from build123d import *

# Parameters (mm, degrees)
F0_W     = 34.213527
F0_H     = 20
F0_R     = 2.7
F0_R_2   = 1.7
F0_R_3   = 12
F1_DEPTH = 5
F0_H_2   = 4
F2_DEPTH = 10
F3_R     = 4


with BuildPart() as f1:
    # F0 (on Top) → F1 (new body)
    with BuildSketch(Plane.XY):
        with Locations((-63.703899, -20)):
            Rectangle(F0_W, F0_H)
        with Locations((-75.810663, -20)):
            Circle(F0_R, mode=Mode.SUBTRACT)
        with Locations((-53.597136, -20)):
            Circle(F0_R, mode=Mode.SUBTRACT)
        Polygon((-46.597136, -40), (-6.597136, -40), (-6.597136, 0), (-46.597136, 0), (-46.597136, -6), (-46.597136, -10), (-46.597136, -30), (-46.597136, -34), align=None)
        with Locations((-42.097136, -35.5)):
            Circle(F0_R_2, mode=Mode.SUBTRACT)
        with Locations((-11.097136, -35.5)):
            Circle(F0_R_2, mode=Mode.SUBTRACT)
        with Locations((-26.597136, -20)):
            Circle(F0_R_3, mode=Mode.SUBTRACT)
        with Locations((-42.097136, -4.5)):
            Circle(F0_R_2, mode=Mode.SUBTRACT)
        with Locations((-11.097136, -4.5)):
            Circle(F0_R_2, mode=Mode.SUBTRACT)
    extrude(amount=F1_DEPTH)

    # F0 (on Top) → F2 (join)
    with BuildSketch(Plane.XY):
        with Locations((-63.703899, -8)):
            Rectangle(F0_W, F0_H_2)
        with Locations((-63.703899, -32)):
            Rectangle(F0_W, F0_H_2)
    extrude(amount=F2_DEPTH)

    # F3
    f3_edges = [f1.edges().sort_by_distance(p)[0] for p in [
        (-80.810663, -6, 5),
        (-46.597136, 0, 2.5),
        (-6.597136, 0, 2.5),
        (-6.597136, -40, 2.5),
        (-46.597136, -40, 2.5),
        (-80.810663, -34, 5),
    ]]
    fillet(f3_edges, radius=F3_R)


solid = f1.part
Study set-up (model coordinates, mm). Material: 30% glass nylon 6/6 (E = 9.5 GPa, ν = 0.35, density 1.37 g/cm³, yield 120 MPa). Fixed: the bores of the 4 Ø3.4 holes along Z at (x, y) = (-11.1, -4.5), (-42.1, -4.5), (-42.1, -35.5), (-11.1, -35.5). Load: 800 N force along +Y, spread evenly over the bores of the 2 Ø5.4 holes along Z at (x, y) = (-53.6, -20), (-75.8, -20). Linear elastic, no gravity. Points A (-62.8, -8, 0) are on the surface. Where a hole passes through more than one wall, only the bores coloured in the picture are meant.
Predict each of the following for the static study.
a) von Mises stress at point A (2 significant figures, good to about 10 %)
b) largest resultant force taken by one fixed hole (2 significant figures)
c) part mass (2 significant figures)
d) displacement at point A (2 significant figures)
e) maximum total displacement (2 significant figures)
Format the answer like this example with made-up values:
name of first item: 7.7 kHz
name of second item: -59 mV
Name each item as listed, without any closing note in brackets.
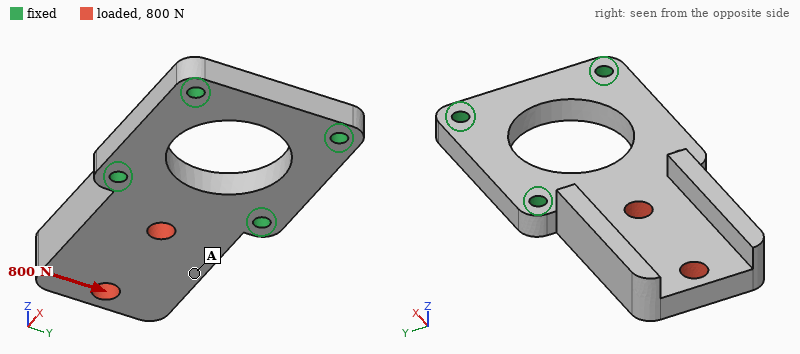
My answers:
von Mises stress at point A: 5.9 MPa
largest resultant force taken by one fixed hole: 710 N
part mass: 16 g
displacement at point A: 0.070 mm
maximum total displacement: 0.12 mm
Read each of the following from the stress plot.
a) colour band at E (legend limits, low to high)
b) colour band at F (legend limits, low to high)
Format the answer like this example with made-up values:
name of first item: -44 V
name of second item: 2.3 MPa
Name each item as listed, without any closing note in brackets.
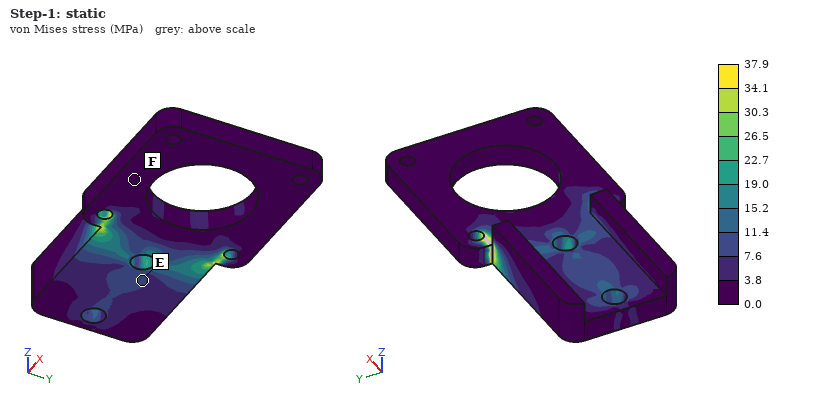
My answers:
colour band at E: 7.6 to 11.4 MPa
colour band at F: 0.0 to 3.8 MPa
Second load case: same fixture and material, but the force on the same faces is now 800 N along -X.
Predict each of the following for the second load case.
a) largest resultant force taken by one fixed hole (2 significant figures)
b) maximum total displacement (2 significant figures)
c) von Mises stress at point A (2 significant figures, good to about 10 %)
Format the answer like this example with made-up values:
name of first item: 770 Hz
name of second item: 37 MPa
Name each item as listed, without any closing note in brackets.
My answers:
largest resultant force taken by one fixed hole: 400 N
maximum total displacement: 47 µm
von Mises stress at point A: 4.1 MPa
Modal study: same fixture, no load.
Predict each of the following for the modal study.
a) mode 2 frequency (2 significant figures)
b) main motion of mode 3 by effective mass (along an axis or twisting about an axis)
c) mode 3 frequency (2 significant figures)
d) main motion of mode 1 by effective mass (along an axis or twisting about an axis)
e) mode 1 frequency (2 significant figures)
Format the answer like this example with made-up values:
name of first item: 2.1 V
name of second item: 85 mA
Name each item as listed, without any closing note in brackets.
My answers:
mode 2 frequency: 3400 Hz
main motion of mode 3 by effective mass: along Y
mode 3 frequency: 5500 Hz
main motion of mode 1 by effective mass: along Z
mode 1 frequency: 1200 Hz
